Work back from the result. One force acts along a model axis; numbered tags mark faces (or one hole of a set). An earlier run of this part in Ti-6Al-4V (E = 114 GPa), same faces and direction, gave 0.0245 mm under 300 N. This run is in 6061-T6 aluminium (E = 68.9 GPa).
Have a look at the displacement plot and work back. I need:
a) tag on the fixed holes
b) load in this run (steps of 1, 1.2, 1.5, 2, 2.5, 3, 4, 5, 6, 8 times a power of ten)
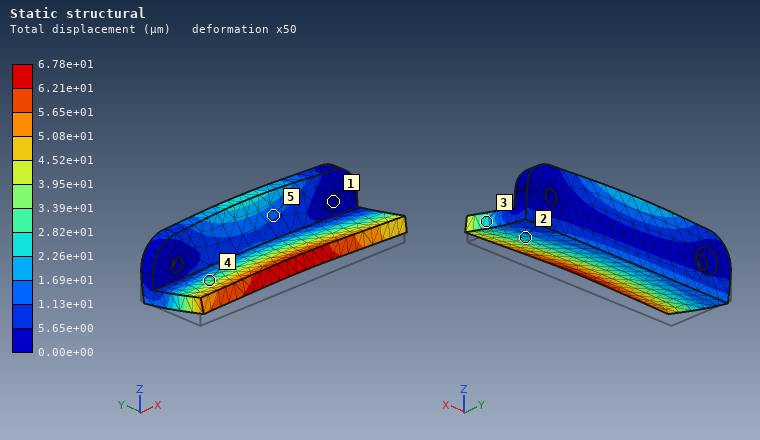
1
500 N
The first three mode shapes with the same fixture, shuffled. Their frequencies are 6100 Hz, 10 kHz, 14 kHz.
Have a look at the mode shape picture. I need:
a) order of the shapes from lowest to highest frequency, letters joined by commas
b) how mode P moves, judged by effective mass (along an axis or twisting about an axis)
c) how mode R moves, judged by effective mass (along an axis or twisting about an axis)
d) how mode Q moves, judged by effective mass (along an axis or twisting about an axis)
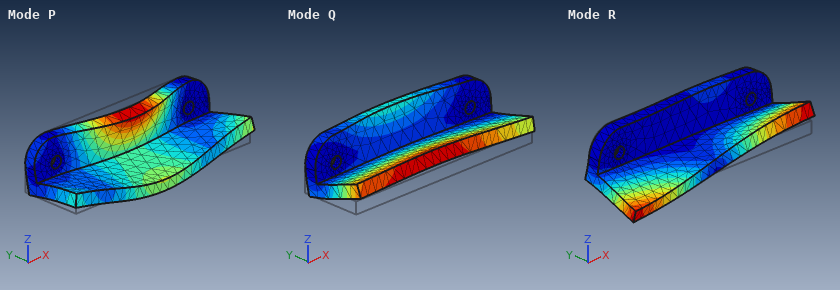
Q, R, P
along Y
twisting about Y
along Z
